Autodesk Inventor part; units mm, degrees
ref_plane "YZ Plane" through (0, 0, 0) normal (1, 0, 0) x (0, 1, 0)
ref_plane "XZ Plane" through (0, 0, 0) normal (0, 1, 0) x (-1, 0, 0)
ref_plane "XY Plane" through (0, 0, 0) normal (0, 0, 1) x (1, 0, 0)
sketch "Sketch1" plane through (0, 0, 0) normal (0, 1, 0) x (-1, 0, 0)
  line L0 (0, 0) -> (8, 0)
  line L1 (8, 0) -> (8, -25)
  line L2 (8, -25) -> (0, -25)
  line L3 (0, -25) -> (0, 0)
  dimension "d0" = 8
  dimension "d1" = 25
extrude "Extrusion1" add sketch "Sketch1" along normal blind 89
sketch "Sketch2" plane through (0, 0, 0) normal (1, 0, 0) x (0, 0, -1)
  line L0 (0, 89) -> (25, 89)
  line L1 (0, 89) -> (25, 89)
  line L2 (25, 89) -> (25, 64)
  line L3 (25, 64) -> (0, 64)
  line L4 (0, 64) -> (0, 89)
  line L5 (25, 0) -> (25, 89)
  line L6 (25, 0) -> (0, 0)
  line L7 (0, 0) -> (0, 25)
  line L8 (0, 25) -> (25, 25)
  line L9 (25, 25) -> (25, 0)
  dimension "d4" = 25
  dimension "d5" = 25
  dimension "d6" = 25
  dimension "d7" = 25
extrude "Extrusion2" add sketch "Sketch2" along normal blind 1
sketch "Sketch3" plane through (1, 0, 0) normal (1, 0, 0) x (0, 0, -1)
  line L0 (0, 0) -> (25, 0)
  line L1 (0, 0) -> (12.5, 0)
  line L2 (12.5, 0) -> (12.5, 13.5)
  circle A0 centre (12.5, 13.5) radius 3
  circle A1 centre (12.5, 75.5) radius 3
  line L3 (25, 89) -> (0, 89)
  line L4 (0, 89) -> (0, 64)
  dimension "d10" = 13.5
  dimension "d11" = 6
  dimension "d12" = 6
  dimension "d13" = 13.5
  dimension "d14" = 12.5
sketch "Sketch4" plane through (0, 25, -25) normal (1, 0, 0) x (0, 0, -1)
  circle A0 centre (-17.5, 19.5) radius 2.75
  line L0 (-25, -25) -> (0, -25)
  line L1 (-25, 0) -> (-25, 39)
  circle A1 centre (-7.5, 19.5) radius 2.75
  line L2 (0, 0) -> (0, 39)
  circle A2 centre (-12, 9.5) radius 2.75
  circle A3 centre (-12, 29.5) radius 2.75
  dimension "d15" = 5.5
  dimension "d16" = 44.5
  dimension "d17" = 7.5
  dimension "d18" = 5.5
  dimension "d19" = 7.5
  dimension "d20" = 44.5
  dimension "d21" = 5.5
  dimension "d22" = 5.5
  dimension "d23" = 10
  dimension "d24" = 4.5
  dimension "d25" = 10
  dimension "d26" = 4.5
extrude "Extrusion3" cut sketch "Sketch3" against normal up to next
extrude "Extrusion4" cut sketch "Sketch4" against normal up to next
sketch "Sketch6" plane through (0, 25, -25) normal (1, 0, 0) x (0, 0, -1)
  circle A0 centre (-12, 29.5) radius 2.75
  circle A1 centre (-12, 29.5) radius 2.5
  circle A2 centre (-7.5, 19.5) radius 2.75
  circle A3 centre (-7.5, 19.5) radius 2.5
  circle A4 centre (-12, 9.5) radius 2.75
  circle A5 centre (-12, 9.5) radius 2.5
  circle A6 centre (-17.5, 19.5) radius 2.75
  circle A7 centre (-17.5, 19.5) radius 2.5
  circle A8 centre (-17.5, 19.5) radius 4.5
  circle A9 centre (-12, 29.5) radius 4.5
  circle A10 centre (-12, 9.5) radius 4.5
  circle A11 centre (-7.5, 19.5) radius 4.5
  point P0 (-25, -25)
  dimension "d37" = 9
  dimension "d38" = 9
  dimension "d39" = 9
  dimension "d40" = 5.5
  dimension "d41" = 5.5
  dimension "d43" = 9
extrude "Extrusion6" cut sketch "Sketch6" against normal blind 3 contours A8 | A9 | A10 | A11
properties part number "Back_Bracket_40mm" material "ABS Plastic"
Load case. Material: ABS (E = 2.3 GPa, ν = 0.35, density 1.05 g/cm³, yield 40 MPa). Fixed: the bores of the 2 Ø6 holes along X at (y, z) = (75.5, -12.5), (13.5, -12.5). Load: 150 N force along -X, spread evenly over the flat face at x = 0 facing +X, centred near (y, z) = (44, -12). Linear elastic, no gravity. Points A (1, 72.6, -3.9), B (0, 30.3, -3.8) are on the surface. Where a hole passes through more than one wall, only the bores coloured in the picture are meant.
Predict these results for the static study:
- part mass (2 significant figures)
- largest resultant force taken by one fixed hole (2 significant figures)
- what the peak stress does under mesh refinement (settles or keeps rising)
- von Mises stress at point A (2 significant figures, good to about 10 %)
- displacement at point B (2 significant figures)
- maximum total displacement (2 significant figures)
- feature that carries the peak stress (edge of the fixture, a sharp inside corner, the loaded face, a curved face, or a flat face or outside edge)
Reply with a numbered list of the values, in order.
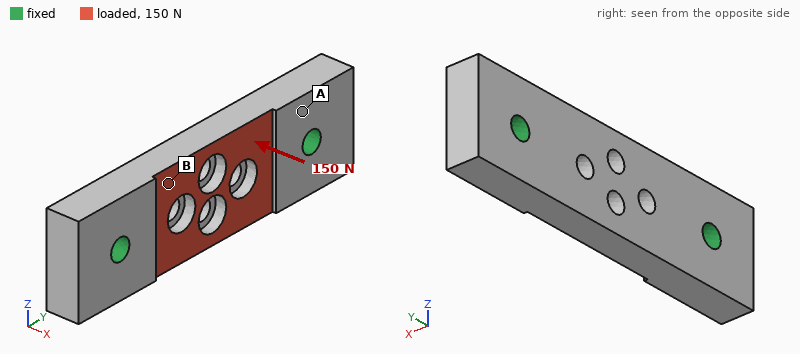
1. 18 g
2. 78 N
3. keeps rising
4. 1.5 MPa
5. 40 µm
6. 67 µm
7. edge of the fixture
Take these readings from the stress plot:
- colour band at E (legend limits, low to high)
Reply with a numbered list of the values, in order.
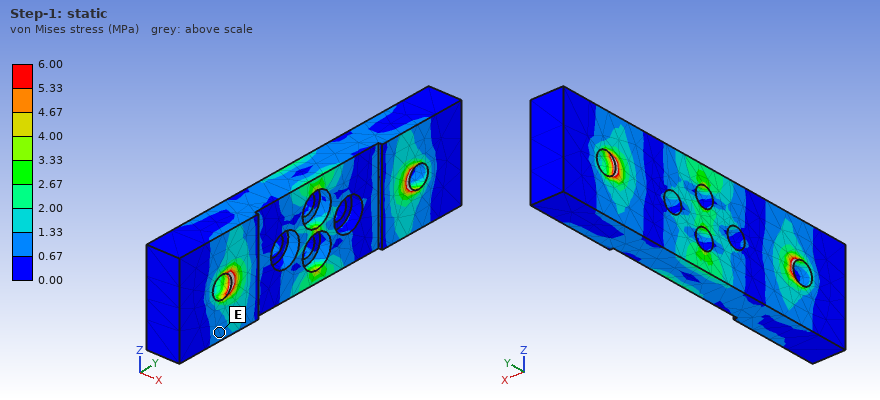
1. 0.67 to 1.33 MPa
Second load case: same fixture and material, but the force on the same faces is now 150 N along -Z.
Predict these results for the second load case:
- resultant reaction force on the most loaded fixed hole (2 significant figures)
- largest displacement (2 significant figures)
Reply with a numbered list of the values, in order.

1. 75 N
2. 39 µm
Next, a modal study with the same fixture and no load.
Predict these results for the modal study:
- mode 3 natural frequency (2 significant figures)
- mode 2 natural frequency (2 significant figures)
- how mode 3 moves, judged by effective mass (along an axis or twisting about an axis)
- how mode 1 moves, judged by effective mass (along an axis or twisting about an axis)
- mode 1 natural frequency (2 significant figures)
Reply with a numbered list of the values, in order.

1. 4700 Hz
2. 4400 Hz
3. along Z
4. along X
5. 3200 Hz
